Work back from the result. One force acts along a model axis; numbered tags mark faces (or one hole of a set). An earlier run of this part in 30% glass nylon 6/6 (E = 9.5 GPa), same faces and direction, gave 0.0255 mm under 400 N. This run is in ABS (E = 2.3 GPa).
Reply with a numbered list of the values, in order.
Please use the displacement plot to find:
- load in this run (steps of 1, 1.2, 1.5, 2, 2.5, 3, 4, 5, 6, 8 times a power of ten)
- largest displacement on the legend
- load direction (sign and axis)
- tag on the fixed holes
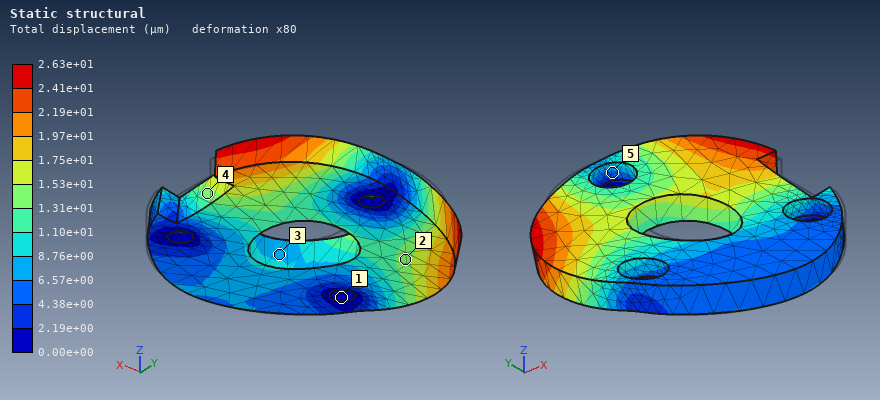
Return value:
1. 100 N
2. 2.63e+01 µm
3. -X
4. 1
